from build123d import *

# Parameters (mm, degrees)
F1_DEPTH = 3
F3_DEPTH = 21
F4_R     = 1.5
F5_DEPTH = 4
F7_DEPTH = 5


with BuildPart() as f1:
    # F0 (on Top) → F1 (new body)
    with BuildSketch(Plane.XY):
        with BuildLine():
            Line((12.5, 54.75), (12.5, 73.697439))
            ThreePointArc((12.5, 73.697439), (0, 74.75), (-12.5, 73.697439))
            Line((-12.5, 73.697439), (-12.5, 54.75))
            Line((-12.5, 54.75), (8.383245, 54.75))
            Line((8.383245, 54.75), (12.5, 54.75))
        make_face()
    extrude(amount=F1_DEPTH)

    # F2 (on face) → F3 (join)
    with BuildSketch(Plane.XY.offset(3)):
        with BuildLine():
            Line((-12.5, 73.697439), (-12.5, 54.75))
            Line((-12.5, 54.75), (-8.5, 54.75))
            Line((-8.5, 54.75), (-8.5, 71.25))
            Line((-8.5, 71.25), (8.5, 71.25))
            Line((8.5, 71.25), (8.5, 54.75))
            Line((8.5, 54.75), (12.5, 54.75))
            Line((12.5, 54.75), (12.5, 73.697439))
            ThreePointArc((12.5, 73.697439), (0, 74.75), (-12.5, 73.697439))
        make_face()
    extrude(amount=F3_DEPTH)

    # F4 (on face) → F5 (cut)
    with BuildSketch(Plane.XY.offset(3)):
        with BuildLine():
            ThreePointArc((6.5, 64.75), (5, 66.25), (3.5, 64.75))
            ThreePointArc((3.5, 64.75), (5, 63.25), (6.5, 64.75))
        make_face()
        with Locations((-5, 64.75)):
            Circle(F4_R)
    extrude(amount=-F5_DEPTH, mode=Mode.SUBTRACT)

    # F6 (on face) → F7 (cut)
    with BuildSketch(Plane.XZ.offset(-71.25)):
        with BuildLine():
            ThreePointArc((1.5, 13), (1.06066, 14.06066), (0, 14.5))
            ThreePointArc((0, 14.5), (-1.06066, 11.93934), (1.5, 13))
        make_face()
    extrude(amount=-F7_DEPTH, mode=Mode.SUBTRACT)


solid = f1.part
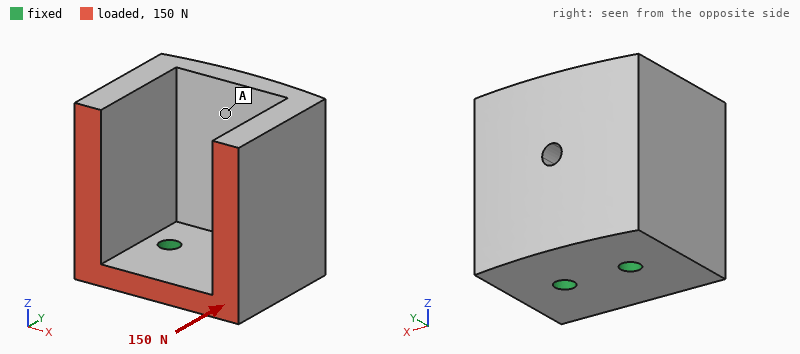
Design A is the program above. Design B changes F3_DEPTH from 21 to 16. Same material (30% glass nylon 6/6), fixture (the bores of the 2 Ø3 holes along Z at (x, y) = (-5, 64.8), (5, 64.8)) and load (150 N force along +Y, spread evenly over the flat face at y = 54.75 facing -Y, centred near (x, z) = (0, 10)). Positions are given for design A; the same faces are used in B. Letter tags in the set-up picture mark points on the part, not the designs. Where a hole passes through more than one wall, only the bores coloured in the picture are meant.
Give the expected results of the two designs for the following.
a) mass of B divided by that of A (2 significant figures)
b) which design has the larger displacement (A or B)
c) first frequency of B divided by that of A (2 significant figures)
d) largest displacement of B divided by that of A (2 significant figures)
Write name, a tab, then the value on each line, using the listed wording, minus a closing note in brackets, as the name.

mass of B divided by that of A	0.82
which design has the larger displacement	A
first frequency of B divided by that of A	1.4
largest displacement of B divided by that of A	0.61
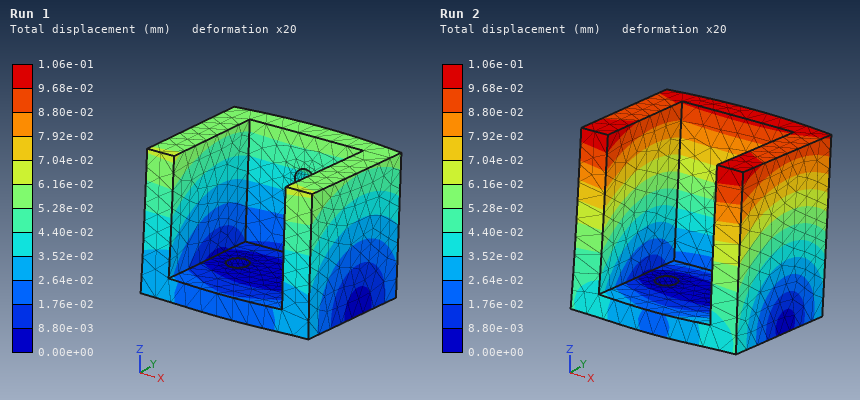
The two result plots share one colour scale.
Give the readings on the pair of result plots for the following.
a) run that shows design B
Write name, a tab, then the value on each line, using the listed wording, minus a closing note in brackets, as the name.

run that shows design B	Run 1
